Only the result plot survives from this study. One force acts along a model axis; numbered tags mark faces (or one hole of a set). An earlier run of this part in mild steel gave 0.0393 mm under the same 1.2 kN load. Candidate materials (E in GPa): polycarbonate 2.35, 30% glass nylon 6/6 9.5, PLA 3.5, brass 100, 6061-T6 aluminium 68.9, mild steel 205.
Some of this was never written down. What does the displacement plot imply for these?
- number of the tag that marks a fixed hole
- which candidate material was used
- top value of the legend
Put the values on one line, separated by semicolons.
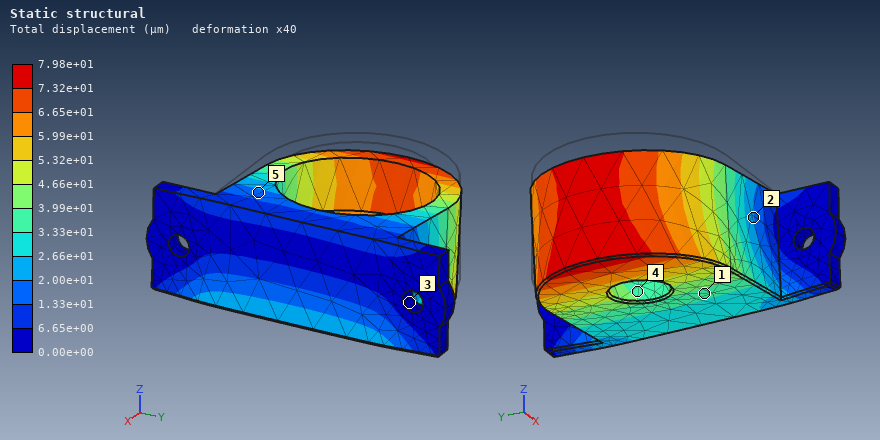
3; brass; 7.98e+01 µm
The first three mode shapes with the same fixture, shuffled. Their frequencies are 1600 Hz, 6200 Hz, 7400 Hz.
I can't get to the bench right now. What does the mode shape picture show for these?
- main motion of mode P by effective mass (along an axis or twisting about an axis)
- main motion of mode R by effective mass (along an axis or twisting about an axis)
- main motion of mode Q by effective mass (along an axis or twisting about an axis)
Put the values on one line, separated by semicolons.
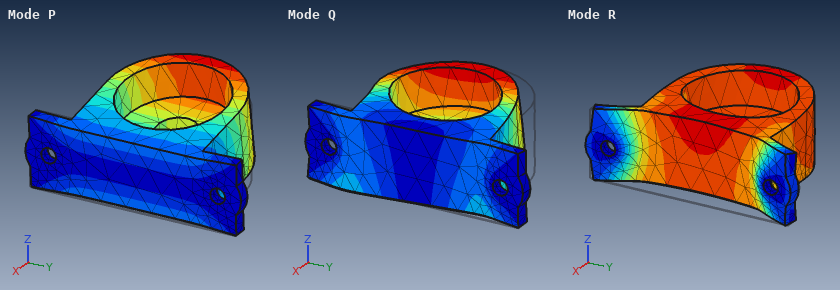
along Z; along X; along Y
